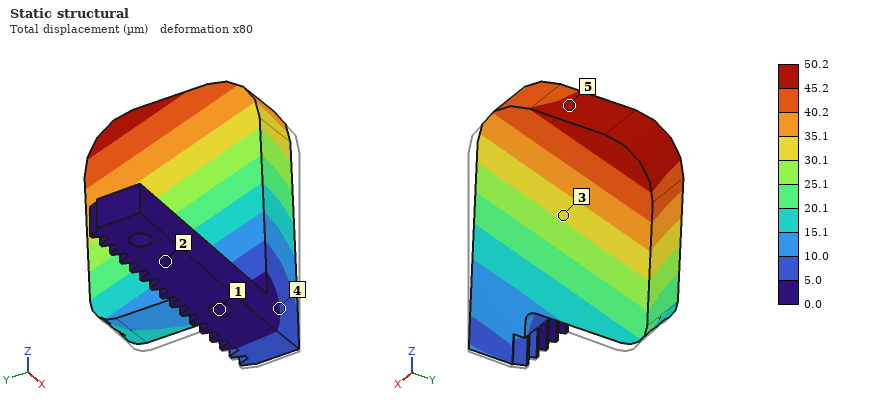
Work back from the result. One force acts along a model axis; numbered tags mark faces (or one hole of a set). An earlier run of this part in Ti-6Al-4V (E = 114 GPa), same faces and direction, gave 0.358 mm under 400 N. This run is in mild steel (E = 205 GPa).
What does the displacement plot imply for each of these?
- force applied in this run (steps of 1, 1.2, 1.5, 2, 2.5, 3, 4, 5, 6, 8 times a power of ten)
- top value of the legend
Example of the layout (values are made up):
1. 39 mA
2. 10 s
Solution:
1. 100 N
2. 50.2 µm
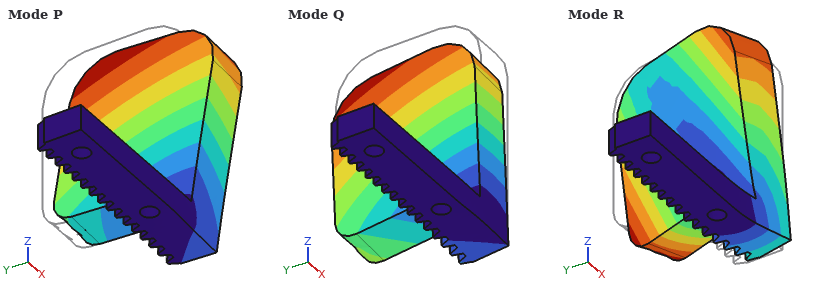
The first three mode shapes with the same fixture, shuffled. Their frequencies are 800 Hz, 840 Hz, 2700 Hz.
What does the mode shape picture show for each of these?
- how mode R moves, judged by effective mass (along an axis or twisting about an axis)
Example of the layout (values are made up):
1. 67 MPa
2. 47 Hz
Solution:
1. twisting about Z
